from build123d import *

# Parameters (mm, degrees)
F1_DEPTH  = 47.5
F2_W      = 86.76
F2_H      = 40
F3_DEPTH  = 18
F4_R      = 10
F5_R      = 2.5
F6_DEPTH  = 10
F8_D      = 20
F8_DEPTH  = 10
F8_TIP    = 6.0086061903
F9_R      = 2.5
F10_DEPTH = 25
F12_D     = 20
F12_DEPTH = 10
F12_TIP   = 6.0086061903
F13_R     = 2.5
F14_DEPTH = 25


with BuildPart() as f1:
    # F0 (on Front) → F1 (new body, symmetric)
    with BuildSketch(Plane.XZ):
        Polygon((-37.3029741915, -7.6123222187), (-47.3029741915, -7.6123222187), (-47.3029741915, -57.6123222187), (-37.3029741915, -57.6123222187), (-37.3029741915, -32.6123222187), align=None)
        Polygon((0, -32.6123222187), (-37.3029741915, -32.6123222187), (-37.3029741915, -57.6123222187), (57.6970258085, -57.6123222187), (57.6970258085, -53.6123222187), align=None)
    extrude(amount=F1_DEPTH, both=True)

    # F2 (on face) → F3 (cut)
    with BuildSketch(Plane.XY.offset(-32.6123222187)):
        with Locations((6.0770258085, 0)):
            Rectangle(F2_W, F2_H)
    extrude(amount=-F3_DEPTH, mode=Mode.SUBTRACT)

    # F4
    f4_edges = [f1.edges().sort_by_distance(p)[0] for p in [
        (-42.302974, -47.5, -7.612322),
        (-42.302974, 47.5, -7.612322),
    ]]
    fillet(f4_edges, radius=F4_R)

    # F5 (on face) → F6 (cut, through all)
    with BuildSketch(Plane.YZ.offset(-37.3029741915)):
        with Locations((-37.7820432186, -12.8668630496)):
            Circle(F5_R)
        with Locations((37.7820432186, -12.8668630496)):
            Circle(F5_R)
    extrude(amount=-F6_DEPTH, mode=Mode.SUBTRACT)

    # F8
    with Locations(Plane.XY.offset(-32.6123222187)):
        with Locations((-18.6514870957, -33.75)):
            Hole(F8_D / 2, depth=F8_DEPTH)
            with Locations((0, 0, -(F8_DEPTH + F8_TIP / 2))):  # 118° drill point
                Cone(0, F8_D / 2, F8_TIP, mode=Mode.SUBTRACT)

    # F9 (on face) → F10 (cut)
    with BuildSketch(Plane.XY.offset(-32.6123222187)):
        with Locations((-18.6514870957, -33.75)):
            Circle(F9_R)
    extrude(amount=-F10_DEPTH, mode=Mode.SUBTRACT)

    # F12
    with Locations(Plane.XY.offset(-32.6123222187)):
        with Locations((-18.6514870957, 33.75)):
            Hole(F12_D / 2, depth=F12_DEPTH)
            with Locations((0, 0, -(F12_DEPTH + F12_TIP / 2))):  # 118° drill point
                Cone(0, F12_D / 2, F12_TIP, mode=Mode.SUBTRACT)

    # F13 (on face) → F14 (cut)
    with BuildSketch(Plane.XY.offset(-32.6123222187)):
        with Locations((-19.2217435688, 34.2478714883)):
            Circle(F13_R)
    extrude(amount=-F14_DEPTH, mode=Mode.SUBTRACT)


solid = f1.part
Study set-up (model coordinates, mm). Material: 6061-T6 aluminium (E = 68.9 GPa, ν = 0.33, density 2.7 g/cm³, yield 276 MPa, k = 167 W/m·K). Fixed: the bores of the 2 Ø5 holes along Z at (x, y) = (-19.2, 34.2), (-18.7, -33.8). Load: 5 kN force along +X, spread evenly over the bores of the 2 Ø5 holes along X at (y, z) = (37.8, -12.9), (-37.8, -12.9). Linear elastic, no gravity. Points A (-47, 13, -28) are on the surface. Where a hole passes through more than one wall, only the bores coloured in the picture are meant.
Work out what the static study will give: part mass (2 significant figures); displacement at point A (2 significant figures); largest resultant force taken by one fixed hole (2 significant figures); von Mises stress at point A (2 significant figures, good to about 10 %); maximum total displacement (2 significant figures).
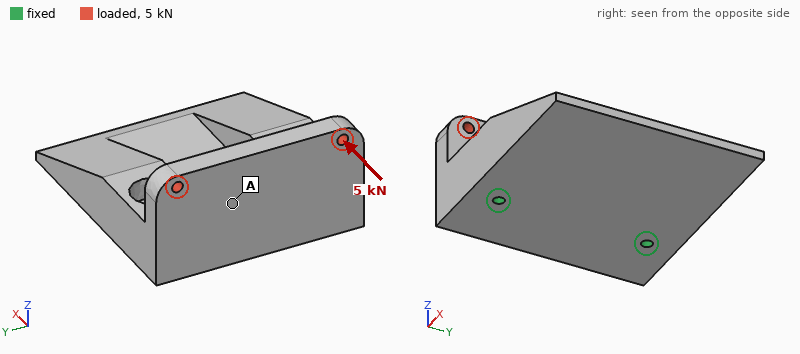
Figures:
440 g
0.14 mm
2.5 kN
32 MPa
0.28 mm
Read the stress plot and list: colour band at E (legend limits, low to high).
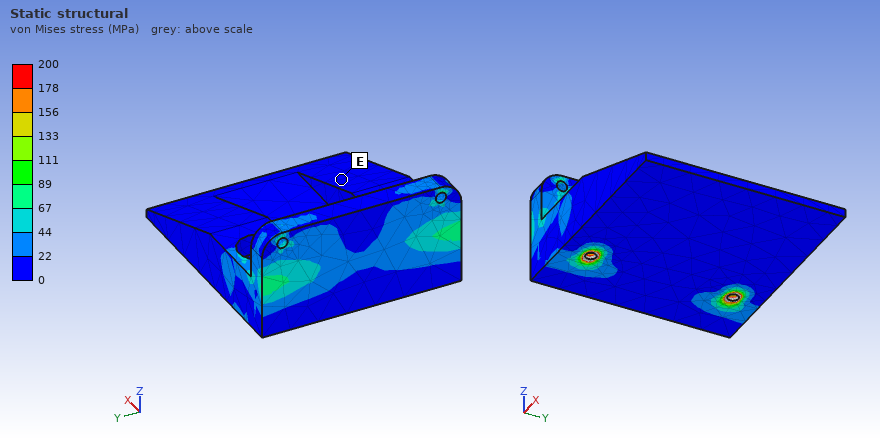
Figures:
0 to 22 MPa
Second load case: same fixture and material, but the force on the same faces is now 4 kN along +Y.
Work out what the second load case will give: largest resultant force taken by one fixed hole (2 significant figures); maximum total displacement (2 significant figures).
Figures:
3.2 kN
49 µm
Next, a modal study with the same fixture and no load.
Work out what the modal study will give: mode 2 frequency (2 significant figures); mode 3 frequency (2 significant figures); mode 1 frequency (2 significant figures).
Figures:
3400 Hz
4400 Hz
1700 Hz
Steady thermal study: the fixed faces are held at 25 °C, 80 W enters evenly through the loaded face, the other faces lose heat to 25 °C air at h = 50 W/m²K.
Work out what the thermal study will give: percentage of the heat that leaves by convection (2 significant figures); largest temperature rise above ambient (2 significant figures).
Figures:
16 %
35 K
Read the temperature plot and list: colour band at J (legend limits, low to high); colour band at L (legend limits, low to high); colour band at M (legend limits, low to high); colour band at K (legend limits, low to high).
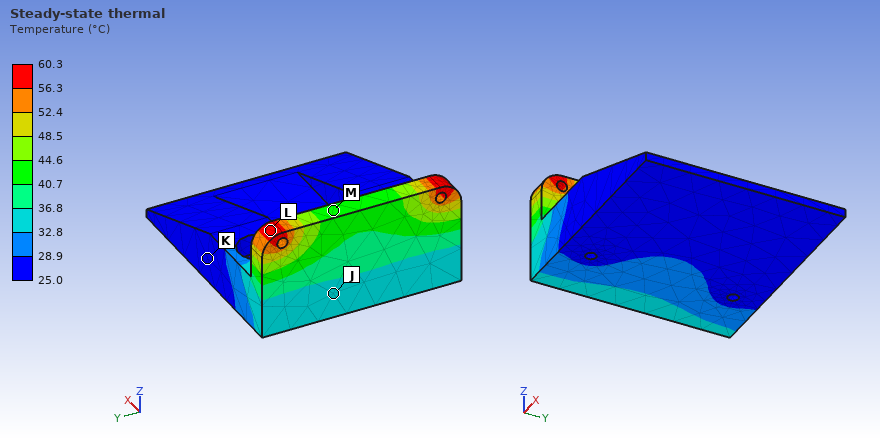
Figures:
32.8 to 36.8 °C
56.3 to 60.3 °C
40.7 to 44.6 °C
25.0 to 28.9 °C
